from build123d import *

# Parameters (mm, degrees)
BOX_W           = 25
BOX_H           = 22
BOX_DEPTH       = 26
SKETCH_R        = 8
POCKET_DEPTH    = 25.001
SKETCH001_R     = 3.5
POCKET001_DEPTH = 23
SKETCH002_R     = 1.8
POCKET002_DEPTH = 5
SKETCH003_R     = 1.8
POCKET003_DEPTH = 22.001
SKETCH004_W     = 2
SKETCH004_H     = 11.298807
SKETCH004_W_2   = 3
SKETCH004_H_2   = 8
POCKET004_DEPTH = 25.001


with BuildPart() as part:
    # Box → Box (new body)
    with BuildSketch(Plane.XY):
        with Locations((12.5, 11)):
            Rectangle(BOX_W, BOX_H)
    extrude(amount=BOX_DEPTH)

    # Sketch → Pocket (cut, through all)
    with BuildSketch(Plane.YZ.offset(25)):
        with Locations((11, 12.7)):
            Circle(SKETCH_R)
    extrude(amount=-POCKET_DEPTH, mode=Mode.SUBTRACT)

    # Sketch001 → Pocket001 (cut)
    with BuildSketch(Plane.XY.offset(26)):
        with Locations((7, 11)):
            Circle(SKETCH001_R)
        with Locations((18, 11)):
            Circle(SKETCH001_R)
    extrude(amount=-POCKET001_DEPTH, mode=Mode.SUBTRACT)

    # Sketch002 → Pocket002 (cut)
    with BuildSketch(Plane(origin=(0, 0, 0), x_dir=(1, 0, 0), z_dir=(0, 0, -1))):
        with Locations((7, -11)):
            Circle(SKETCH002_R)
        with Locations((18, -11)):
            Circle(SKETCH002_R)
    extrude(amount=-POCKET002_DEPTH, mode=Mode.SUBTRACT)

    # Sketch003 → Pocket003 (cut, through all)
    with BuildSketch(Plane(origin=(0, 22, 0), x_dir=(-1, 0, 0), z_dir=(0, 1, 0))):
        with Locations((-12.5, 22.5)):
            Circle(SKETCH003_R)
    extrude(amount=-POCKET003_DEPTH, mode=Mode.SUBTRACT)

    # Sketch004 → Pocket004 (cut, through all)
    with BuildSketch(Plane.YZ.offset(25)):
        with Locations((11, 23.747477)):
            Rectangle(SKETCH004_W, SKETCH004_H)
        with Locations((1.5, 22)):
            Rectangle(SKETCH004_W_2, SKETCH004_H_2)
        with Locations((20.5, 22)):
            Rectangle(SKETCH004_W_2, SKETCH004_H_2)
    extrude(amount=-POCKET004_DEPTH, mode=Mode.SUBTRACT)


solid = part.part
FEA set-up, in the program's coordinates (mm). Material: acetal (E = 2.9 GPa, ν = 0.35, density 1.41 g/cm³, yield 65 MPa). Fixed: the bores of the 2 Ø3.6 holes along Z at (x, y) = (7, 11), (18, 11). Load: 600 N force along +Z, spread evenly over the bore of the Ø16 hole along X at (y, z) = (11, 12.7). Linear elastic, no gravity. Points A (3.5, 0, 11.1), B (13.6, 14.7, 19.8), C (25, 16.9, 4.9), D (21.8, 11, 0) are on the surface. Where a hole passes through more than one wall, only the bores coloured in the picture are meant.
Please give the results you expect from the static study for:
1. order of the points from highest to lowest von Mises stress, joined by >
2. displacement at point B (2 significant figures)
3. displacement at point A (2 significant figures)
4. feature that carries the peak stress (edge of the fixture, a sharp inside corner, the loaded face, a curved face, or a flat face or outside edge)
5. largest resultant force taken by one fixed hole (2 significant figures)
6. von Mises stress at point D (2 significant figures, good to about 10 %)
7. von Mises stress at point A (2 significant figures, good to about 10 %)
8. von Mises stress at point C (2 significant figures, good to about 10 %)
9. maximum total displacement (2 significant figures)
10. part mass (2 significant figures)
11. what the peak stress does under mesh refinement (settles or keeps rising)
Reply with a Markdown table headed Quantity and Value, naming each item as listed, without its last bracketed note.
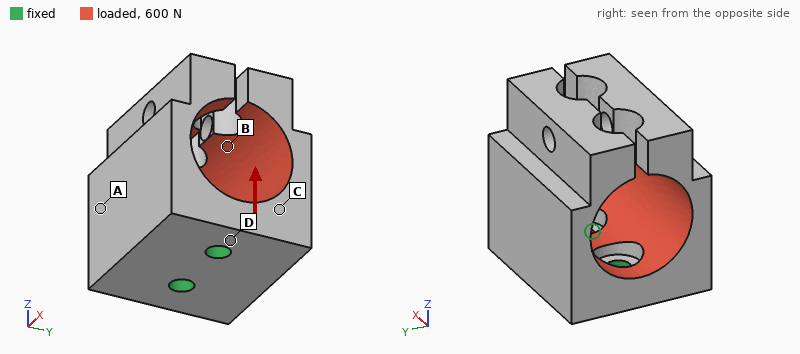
| Quantity | Value |
|---|---|
| order of the points from highest to lowest von Mises stress, joined by > | D > A > C > B |
| displacement at point B | 0.23 mm |
| displacement at point A | 0.099 mm |
| feature that carries the peak stress | edge of the fixture |
| largest resultant force taken by one fixed hole | 300 N |
| von Mises stress at point D | 13 MPa |
| von Mises stress at point A | 9.7 MPa |
| von Mises stress at point C | 4.6 MPa |
| maximum total displacement | 0.39 mm |
| part mass | 10 g |
| what the peak stress does under mesh refinement | keeps rising |
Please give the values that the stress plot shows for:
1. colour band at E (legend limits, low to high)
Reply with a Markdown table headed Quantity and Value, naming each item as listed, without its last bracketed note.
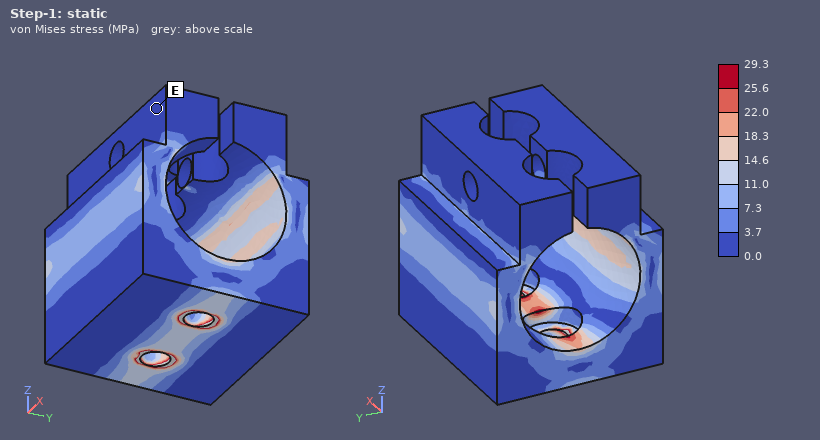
| Quantity | Value |
|---|---|
| colour band at E | 0.0 to 3.7 MPa |
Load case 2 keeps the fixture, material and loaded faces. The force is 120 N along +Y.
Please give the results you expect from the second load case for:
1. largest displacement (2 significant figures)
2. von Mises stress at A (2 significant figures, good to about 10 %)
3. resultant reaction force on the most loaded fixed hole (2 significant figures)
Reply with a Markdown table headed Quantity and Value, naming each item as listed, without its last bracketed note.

| Quantity | Value |
|---|---|
| largest displacement | 0.41 mm |
| von Mises stress at A | 3.9 MPa |
| resultant reaction force on the most loaded fixed hole | 60 N |
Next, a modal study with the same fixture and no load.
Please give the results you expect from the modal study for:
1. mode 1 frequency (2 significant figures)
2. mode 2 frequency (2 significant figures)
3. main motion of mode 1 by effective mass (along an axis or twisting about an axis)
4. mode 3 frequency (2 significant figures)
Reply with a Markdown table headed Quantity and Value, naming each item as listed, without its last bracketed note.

| Quantity | Value |
|---|---|
| mode 1 frequency | 1000 Hz |
| mode 2 frequency | 1200 Hz |
| main motion of mode 1 by effective mass | along Y |
| mode 3 frequency | 2000 Hz |
